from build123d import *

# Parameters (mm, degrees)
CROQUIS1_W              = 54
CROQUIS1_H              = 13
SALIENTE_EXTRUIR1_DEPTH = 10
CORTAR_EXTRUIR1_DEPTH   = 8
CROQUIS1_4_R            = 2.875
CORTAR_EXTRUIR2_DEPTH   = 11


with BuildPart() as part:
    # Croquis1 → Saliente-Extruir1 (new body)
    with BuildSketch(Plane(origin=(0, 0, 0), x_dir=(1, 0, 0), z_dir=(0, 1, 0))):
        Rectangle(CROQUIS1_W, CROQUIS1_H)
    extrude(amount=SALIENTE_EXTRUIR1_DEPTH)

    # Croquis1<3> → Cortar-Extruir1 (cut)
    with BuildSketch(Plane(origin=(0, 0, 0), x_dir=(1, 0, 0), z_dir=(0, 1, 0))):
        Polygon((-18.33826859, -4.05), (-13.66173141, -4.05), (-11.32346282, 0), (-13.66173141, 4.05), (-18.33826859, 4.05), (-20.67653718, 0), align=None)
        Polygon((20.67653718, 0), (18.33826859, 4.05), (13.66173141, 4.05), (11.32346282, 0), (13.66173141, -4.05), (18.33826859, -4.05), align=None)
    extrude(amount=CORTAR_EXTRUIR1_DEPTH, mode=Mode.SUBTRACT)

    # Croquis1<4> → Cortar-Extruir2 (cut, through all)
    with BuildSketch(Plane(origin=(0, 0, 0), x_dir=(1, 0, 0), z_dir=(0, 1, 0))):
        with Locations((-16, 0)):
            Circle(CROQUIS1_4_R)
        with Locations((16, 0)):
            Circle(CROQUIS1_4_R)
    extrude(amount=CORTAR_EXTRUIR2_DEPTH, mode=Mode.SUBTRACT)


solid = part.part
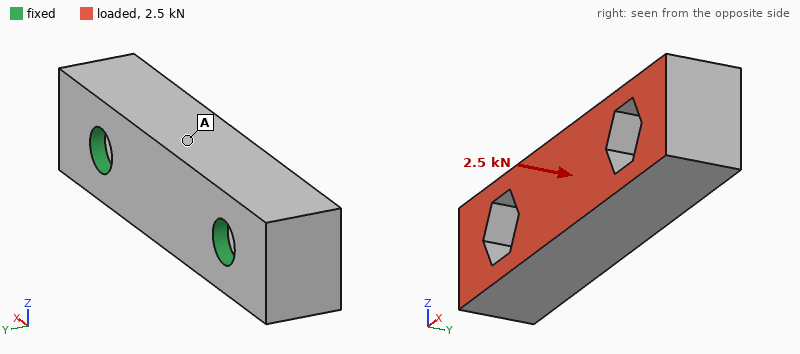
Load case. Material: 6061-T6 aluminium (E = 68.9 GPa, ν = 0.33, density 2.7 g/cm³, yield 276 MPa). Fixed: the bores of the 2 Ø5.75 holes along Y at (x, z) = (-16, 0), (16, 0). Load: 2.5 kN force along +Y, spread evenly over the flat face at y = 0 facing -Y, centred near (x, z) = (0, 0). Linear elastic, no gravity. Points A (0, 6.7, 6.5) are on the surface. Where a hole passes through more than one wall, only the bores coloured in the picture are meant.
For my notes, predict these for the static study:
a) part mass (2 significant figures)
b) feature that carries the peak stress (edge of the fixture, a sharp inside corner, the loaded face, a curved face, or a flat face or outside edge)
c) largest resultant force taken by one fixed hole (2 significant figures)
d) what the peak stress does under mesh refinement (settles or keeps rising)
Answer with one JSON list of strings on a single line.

["16 g", "edge of the fixture", "1.3 kN", "keeps rising"]
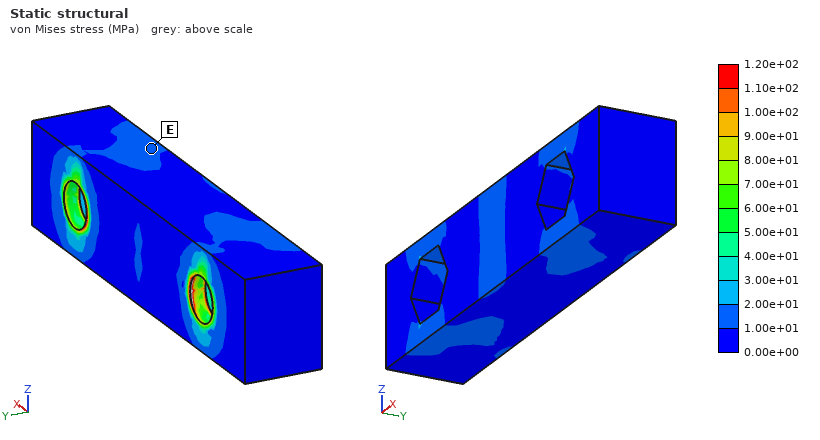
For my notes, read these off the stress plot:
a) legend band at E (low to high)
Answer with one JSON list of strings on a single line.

["1.00e+01 to 2.00e+01 MPa"]
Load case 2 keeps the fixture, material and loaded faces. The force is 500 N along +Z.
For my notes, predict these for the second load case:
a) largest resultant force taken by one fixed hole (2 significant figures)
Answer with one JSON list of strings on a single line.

["250 N"]
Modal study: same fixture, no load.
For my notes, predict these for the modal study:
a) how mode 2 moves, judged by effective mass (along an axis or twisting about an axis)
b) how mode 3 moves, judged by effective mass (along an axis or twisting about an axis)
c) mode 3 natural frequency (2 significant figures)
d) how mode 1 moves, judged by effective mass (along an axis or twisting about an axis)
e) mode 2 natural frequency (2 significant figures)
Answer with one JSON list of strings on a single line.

["twisting about Y", "along Y", "23 kHz", "along Z", "21 kHz"]
